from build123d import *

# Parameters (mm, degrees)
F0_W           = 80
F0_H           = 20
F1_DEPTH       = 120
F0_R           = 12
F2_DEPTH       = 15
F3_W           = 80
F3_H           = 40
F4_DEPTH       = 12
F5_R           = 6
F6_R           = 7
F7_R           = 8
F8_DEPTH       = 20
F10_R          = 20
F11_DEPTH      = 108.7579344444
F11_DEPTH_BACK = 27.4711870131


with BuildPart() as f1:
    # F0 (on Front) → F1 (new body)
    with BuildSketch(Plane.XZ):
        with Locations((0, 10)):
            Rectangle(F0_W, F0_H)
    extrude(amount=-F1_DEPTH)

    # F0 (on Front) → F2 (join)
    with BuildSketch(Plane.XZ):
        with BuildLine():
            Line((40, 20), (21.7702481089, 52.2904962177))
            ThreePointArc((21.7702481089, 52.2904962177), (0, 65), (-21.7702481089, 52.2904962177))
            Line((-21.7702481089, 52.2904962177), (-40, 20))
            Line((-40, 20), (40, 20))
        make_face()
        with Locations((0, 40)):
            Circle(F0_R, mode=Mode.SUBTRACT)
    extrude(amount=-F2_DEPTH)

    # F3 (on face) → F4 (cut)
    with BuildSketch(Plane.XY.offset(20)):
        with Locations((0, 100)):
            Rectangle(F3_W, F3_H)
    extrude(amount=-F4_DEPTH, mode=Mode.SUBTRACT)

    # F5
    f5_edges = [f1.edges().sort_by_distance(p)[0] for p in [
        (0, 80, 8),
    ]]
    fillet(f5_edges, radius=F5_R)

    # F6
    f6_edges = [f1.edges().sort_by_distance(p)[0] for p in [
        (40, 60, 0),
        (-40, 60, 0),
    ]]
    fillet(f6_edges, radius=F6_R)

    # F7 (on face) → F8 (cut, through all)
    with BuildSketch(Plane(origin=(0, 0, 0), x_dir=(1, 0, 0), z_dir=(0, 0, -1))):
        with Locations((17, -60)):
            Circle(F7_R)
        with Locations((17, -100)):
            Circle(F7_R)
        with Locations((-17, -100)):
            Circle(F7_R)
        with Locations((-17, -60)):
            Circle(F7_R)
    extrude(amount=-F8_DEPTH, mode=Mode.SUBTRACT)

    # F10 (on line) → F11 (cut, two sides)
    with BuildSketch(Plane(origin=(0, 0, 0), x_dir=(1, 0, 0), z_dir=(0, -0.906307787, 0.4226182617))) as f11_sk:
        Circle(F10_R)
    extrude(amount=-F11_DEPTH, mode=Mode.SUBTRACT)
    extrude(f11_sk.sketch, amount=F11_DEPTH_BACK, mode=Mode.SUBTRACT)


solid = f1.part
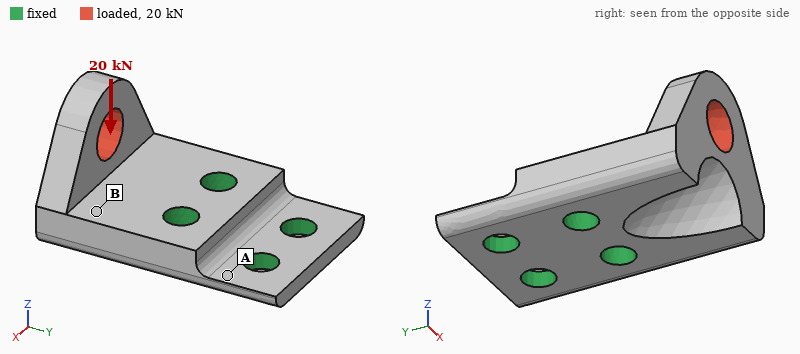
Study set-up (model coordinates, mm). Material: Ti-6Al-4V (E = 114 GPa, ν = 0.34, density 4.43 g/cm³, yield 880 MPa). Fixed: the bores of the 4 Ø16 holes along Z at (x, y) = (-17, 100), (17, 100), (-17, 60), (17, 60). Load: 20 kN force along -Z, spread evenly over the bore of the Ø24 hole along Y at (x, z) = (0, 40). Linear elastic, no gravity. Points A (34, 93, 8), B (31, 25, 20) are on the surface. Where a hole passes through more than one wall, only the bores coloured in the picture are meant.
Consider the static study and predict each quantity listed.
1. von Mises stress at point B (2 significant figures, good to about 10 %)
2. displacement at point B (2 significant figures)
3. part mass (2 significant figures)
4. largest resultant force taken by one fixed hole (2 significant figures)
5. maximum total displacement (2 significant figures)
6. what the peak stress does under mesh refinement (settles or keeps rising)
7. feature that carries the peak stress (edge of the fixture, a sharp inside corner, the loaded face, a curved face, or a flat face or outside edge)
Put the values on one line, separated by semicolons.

80 MPa; 0.081 mm; 690 g; 11 kN; 0.33 mm; keeps rising; edge of the fixture
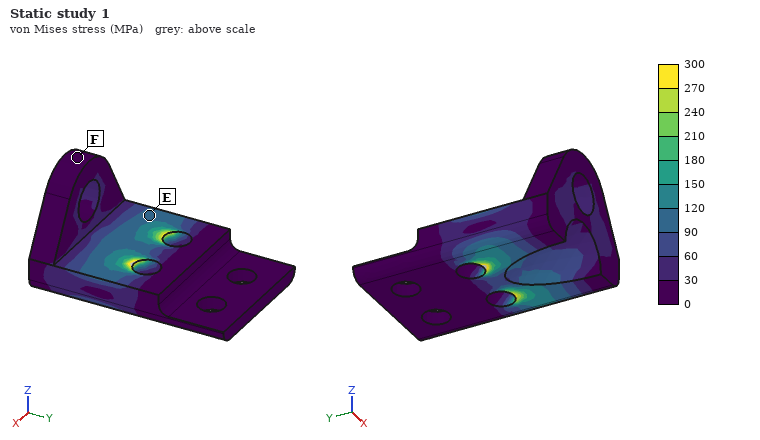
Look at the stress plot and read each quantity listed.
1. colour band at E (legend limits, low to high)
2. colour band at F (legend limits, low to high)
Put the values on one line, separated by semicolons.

90 to 120 MPa; 0 to 30 MPa
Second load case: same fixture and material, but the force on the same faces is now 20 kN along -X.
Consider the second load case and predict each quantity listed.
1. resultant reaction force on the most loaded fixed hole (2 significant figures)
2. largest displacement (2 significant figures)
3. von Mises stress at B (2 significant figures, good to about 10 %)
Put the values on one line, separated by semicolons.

23 kN; 0.20 mm; 86 MPa
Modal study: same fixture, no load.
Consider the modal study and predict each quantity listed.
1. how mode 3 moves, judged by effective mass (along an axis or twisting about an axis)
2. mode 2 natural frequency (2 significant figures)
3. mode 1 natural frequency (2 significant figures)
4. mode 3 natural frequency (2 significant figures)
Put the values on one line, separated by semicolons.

along Z; 4300 Hz; 2900 Hz; 6000 Hz
